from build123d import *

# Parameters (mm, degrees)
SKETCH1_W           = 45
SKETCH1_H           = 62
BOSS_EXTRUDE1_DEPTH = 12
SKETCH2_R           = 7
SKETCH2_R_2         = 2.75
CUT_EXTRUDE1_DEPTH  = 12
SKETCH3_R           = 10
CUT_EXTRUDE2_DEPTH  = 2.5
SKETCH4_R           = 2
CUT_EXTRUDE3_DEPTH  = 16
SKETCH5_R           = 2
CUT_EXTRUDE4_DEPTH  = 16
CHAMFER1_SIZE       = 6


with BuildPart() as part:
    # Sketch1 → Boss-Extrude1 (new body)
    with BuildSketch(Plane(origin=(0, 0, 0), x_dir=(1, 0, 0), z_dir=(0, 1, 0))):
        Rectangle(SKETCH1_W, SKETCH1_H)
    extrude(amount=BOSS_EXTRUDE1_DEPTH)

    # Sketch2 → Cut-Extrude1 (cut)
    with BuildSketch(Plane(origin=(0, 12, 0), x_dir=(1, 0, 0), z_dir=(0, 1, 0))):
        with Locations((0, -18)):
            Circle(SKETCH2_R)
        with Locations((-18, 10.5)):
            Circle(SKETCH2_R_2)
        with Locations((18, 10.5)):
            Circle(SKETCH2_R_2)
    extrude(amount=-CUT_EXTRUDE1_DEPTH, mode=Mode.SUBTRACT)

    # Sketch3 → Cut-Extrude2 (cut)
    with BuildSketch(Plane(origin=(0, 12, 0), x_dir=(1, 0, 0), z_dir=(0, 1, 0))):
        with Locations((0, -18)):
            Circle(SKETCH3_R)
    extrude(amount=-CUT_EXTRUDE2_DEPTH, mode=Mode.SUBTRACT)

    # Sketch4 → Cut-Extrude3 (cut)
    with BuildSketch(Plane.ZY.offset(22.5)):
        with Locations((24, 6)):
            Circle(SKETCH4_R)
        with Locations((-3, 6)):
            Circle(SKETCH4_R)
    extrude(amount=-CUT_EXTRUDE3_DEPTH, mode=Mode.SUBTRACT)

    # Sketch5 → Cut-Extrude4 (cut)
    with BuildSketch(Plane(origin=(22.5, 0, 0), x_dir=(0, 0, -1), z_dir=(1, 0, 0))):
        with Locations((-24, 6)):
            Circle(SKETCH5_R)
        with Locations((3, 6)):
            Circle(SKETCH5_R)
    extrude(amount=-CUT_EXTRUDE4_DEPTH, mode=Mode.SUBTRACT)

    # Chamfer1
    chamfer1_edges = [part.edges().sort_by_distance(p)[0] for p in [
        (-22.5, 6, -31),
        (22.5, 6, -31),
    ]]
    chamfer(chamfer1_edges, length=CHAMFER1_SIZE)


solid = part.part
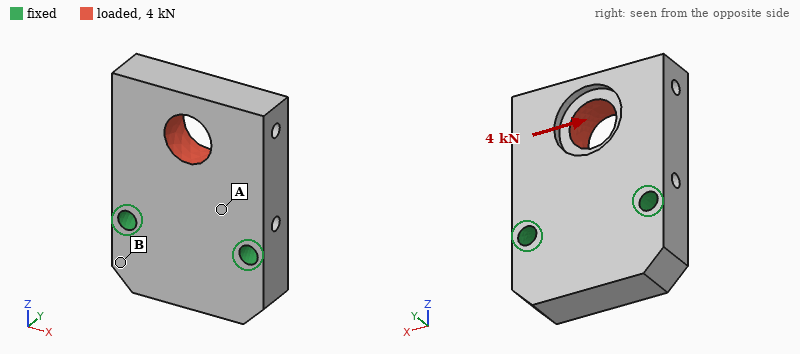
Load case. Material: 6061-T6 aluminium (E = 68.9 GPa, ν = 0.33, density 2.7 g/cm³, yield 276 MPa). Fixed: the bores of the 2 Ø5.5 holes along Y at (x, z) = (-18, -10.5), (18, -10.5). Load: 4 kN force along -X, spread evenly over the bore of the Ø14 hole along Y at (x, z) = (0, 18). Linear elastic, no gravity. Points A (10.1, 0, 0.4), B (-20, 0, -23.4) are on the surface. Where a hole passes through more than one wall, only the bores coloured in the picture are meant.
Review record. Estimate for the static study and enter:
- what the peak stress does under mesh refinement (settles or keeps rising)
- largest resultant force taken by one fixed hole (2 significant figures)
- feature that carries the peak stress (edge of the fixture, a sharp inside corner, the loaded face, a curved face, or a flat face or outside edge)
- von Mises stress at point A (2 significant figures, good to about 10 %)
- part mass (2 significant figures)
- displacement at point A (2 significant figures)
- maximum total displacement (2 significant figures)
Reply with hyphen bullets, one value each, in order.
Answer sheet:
- keeps rising
- 3.6 kN
- edge of the fixture
- 21 MPa
- 79 g
- 5.1 µm
- 29 µm
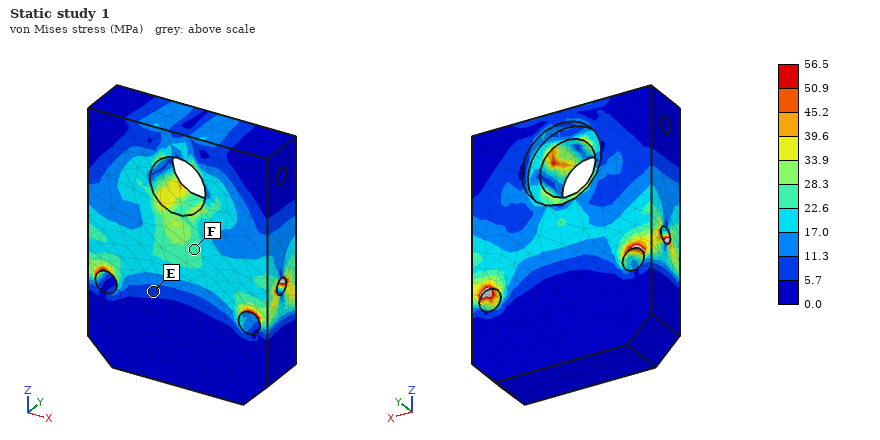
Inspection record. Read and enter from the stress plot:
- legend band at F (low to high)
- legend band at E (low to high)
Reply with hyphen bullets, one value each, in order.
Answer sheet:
- 22.6 to 28.3 MPa
- 5.7 to 11.3 MPa
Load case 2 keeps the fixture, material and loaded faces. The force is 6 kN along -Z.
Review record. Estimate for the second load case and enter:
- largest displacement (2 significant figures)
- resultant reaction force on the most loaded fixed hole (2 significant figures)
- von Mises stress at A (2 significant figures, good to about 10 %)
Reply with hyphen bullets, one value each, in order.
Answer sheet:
- 23 µm
- 3.0 kN
- 22 MPa
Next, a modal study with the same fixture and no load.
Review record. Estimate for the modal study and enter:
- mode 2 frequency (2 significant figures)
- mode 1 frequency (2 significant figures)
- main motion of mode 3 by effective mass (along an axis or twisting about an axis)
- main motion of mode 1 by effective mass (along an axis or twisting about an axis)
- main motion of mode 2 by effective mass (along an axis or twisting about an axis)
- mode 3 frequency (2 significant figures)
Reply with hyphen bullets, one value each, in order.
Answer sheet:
- 9900 Hz
- 5200 Hz
- along X
- along Y
- twisting about Z
- 12 kHz
